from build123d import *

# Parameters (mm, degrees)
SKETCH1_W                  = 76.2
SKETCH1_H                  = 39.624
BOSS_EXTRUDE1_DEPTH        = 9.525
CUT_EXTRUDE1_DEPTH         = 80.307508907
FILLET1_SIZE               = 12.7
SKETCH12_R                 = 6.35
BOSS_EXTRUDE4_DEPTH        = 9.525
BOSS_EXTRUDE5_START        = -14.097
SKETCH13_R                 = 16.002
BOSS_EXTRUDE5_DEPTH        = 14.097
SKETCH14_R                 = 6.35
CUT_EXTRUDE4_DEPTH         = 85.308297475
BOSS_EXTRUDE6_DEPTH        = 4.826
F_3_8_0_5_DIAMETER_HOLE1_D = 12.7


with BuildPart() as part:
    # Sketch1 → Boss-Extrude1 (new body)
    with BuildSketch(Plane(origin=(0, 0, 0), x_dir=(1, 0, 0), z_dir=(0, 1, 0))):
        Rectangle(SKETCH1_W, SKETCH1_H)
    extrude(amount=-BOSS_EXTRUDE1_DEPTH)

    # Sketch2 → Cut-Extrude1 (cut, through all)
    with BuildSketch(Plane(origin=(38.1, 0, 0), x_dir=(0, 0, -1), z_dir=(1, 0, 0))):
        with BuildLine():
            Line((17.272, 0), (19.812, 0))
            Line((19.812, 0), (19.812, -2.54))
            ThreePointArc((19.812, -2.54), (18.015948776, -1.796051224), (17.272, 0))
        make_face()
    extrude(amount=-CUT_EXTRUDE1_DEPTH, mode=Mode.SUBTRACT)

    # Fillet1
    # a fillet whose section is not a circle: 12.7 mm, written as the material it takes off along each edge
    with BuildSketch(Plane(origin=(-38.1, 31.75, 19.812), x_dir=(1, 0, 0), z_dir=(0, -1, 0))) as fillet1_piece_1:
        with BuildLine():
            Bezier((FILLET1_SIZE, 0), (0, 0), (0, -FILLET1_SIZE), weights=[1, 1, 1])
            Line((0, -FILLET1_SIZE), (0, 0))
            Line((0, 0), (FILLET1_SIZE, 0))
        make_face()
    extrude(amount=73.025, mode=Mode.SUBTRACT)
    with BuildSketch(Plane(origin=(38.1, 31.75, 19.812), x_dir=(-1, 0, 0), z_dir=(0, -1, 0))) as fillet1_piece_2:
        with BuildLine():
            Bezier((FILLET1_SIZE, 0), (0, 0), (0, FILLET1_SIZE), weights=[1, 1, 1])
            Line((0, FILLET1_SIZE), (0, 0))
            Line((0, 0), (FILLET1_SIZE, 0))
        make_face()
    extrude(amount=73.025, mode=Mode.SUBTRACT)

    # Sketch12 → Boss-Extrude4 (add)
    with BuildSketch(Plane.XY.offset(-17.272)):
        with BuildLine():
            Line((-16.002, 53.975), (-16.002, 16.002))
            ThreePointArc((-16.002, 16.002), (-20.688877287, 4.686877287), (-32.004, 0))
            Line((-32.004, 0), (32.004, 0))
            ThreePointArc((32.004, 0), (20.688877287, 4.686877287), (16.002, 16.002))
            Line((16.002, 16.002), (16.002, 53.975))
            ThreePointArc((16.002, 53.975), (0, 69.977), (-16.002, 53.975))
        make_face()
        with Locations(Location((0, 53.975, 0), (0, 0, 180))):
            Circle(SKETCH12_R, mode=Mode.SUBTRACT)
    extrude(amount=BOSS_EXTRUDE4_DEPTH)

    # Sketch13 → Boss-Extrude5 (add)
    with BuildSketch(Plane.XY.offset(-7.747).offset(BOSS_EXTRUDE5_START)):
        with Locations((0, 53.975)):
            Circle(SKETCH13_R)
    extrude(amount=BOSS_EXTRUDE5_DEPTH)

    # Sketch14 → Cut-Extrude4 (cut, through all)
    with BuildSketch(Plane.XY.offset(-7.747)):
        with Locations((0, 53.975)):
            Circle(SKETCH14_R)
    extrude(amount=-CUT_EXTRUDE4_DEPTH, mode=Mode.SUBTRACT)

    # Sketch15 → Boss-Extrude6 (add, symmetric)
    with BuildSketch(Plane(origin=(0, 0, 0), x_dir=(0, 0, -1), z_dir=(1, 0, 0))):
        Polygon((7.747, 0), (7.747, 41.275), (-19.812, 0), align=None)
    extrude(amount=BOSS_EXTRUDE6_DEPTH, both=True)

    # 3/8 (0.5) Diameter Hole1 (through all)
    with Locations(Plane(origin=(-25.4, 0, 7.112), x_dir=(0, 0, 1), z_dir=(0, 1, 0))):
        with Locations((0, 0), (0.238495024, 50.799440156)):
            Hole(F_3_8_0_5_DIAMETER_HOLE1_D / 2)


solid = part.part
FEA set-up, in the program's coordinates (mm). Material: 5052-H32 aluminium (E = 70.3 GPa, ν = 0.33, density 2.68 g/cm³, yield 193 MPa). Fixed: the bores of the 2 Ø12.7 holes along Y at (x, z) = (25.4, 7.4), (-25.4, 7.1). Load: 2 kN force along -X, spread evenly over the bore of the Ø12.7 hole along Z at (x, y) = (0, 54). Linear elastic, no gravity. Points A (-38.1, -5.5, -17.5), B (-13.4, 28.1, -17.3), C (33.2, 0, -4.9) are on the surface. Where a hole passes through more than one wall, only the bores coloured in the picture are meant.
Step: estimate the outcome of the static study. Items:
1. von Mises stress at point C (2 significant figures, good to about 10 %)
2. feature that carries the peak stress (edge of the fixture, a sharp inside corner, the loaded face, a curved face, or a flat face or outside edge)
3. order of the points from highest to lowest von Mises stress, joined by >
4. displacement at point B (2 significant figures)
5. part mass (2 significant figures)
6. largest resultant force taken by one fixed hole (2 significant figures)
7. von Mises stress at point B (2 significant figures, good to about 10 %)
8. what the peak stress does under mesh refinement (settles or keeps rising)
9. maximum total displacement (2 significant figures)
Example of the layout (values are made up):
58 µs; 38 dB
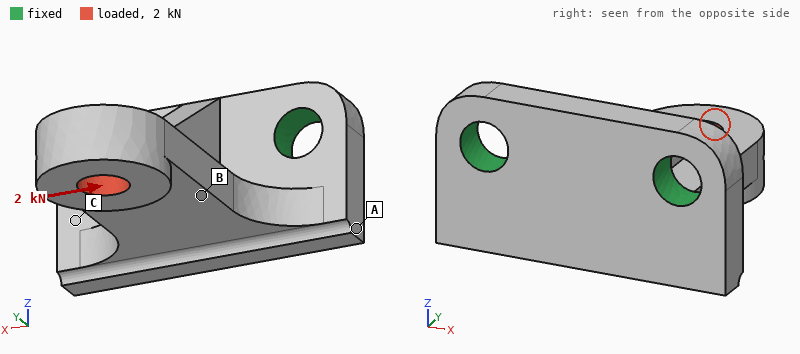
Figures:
17 MPa; edge of the fixture; B > C > A; 0.052 mm; 150 g; 2.9 kN; 30 MPa; keeps rising; 0.15 mm
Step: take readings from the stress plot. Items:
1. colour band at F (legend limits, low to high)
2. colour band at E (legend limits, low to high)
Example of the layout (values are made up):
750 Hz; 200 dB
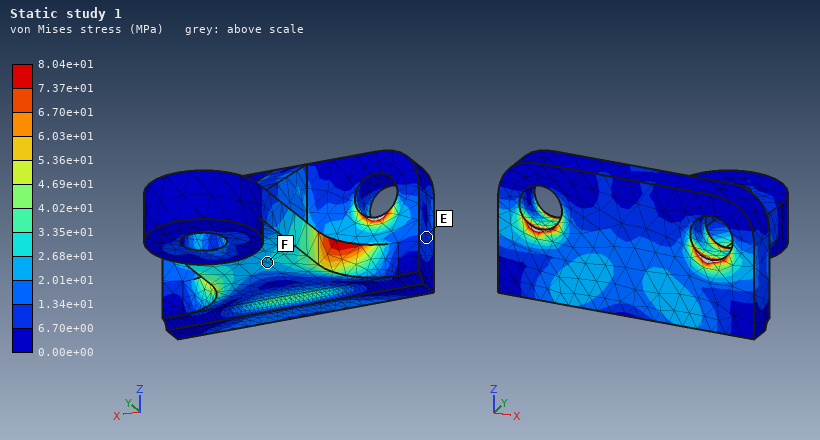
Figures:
2.01e+01 to 2.68e+01 MPa; 6.70e+00 to 1.34e+01 MPa
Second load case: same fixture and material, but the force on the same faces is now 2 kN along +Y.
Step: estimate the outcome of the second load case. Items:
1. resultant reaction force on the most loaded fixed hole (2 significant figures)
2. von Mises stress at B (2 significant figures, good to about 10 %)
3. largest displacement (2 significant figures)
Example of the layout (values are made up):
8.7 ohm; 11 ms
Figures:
1.0 kN; 13 MPa; 83 µm
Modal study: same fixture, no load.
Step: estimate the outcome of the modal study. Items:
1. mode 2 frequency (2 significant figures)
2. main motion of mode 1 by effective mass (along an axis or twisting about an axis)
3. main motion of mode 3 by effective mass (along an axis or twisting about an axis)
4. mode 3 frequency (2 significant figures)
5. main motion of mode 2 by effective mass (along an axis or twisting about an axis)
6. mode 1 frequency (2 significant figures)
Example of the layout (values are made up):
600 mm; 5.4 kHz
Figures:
3700 Hz; along Z; along Y; 7400 Hz; along X; 2300 Hz
